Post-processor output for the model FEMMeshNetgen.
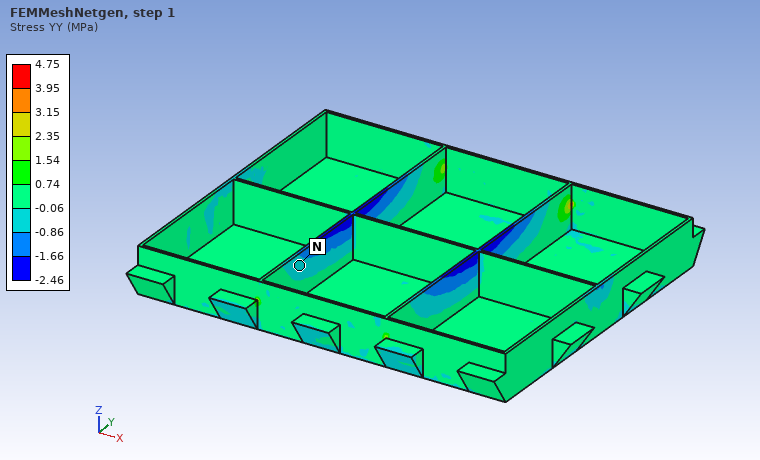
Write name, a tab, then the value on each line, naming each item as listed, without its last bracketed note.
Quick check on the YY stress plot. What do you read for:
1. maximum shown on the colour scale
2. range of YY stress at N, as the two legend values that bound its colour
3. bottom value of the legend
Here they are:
maximum shown on the colour scale	4.75 MPa
range of YY stress at N, as the two legend values that bound its colour	-0.86 to -0.06 MPa
bottom value of the legend	-2.46 MPa
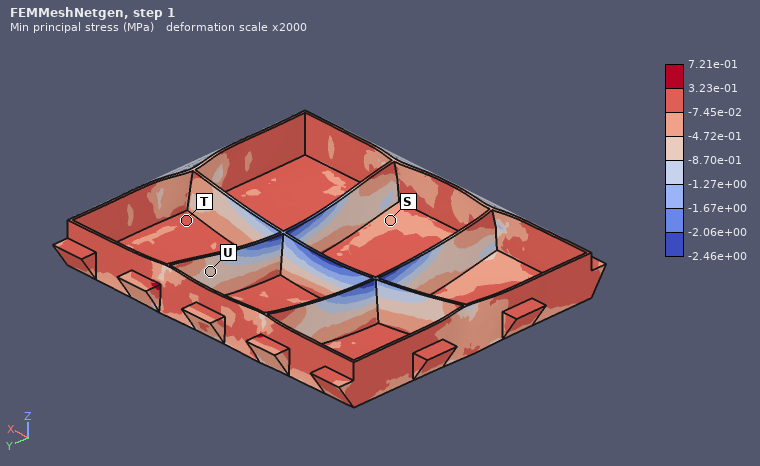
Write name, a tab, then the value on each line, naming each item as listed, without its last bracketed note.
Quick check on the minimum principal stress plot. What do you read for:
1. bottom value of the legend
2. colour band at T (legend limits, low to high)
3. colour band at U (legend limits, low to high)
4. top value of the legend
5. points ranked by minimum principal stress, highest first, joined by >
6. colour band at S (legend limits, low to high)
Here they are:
bottom value of the legend	-2.46e+00 MPa
colour band at T	-7.45e-02 to 3.23e-01 MPa
colour band at U	-8.70e-01 to -4.72e-01 MPa
top value of the legend	7.21e-01 MPa
points ranked by minimum principal stress, highest first, joined by >	T > S > U
colour band at S	-4.72e-01 to -7.45e-02 MPa
